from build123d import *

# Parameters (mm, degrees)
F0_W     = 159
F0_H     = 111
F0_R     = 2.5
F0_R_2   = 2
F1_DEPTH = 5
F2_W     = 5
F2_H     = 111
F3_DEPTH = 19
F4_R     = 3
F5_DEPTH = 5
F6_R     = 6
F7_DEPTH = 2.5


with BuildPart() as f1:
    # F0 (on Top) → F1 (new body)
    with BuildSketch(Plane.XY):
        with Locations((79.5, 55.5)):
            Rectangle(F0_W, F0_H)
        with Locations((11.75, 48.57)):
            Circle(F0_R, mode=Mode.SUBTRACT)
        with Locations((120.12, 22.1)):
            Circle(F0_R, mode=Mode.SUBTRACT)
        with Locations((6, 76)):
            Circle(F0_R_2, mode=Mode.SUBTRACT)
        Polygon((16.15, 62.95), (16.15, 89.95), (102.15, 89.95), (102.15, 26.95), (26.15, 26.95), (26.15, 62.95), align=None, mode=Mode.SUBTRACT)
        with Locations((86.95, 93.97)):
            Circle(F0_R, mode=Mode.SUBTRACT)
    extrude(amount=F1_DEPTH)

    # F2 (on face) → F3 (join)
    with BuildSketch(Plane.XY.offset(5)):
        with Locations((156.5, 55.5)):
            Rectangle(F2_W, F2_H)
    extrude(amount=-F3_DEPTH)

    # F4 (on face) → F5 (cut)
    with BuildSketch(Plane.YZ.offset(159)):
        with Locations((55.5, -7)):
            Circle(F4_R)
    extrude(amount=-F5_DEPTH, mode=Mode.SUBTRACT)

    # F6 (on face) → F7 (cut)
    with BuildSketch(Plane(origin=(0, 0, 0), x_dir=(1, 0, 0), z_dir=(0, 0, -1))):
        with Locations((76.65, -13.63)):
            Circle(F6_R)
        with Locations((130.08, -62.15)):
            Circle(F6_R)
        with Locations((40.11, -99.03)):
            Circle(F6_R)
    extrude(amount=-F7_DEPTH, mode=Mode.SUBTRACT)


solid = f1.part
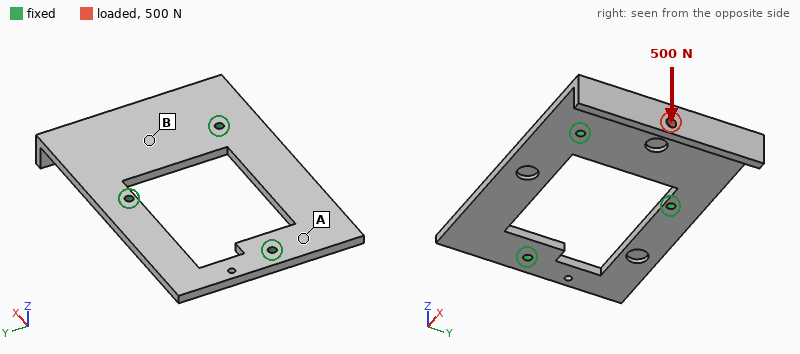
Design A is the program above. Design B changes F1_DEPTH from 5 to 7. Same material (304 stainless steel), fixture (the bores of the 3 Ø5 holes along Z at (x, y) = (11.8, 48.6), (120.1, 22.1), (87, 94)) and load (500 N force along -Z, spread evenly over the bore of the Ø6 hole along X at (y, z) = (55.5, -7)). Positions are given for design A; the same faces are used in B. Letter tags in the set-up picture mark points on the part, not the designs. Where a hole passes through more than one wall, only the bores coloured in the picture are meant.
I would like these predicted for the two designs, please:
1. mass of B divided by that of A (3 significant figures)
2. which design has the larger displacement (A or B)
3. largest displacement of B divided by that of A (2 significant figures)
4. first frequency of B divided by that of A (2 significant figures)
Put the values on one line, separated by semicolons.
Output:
1.36; A; 0.39; 1.4
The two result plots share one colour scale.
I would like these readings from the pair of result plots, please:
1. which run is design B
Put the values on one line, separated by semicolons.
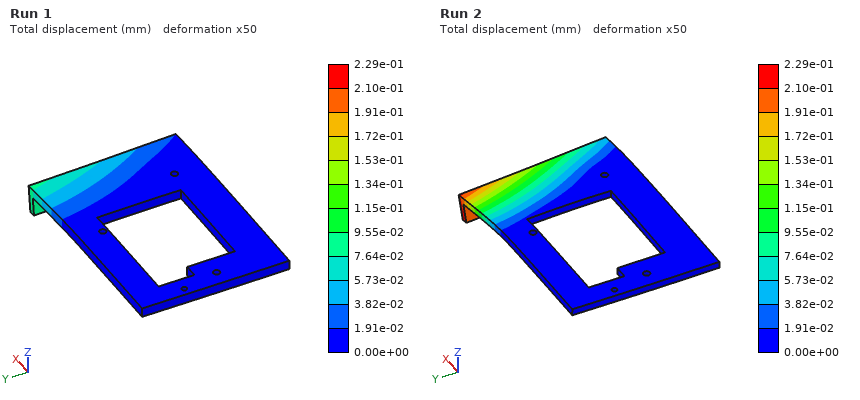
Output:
Run 1
